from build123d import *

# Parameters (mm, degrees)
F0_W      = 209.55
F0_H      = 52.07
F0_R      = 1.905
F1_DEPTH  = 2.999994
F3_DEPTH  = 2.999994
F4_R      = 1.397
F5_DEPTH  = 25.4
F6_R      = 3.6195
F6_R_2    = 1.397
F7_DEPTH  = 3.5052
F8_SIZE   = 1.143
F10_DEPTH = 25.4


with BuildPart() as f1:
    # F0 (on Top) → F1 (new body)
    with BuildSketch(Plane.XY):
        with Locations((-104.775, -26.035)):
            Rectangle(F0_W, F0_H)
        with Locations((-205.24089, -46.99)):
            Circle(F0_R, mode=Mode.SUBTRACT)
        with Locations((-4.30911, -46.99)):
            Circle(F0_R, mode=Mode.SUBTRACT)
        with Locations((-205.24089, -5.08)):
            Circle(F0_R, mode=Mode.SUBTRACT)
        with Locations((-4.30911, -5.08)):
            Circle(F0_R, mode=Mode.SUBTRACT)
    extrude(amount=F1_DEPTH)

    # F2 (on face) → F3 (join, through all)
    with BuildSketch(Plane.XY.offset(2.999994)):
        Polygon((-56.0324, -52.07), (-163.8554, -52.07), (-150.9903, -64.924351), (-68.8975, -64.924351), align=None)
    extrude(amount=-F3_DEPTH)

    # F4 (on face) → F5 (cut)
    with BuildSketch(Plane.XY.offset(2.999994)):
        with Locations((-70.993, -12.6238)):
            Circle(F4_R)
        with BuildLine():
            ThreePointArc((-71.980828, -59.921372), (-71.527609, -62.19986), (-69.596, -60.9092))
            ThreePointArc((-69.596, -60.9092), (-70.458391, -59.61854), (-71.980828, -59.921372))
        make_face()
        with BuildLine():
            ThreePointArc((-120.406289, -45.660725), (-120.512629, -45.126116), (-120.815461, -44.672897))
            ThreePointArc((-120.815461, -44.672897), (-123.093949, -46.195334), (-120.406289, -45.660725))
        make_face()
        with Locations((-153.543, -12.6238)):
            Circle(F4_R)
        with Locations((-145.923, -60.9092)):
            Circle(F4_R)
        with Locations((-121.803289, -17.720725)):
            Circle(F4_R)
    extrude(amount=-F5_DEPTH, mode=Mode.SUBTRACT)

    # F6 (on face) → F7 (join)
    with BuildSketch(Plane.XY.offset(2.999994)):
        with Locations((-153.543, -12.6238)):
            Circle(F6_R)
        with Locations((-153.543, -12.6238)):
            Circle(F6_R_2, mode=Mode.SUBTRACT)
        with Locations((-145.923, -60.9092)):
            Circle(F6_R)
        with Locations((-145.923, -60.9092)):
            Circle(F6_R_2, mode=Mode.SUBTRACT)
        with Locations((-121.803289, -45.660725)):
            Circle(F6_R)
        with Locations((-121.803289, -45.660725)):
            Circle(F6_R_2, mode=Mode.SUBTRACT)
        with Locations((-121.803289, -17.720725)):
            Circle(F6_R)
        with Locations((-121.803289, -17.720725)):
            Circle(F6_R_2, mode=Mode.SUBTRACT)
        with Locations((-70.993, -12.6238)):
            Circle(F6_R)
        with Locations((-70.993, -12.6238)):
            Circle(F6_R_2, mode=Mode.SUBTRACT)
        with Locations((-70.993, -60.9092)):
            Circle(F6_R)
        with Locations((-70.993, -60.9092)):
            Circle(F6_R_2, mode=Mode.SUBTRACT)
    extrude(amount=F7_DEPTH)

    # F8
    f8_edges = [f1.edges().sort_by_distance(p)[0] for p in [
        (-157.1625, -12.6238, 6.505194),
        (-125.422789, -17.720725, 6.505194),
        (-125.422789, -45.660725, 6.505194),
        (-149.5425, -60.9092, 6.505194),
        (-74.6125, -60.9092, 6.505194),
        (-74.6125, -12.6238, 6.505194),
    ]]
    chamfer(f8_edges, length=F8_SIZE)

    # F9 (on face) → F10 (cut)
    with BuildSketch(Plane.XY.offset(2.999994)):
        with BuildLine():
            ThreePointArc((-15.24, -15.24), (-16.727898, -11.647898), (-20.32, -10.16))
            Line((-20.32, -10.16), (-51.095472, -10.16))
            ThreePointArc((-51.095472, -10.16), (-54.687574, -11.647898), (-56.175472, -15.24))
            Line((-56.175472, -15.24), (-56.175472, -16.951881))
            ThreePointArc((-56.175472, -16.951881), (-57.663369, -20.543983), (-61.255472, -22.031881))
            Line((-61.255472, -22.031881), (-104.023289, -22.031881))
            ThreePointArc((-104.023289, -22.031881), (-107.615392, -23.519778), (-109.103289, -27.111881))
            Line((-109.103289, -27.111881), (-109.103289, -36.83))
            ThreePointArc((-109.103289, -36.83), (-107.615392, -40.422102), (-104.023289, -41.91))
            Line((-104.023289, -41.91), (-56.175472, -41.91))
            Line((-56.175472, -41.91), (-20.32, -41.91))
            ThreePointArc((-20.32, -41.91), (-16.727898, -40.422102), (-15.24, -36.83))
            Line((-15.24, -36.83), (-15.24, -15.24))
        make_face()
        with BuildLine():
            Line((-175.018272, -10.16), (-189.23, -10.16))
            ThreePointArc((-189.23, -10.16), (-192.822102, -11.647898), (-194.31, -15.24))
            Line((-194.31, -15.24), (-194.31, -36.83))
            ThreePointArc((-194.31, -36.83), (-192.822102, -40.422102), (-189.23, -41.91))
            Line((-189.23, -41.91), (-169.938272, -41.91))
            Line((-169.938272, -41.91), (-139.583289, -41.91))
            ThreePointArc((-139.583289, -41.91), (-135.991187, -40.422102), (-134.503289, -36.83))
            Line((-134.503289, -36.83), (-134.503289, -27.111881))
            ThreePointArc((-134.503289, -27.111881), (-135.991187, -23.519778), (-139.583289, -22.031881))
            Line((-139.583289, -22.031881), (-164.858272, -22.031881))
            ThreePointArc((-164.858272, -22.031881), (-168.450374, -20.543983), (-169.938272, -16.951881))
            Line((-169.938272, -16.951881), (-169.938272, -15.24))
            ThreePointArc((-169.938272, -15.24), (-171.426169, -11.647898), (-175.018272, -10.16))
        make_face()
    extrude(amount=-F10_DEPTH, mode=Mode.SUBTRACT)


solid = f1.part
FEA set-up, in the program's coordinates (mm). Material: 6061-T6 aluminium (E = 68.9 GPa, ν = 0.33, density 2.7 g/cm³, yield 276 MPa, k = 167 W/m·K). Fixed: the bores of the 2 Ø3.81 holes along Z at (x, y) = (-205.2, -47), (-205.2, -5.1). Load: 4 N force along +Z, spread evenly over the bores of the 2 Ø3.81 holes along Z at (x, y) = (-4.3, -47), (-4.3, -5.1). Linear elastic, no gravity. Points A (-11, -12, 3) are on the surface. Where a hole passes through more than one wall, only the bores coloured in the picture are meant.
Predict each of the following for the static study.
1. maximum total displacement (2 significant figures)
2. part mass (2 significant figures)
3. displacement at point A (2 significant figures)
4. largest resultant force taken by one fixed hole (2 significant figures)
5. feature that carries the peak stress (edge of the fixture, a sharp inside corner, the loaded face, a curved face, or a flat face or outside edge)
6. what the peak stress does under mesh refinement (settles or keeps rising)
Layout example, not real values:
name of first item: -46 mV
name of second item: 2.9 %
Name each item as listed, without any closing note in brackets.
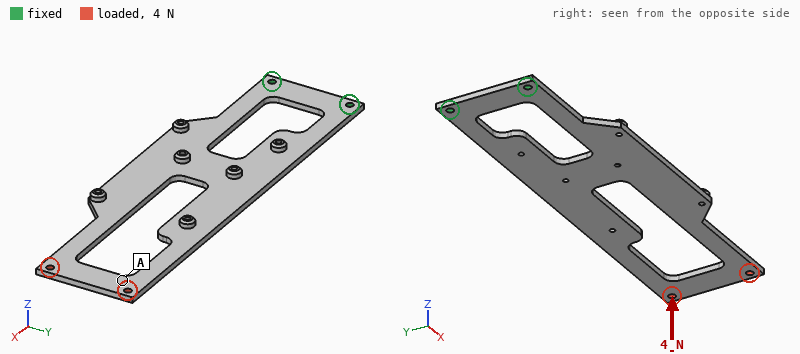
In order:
maximum total displacement: 2.4 mm
part mass: 69 g
displacement at point A: 2.2 mm
largest resultant force taken by one fixed hole: 2.1 N
feature that carries the peak stress: edge of the fixture
what the peak stress does under mesh refinement: keeps rising
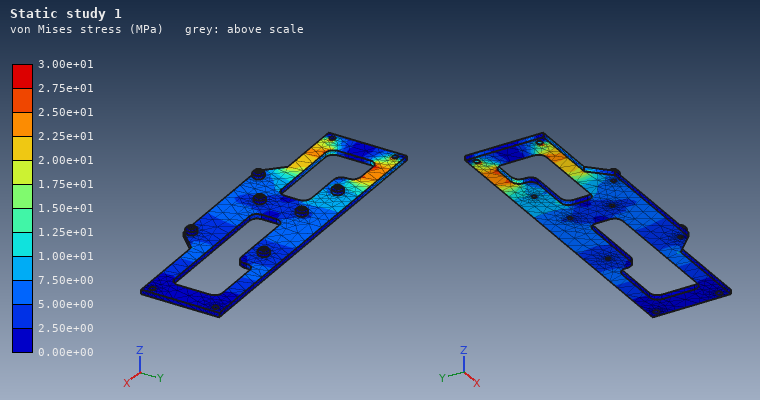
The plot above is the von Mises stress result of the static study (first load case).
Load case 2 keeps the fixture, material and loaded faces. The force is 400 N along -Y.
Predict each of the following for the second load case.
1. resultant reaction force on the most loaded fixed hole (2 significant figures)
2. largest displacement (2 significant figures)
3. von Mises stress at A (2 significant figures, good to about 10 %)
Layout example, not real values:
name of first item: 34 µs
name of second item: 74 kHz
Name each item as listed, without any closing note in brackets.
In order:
resultant reaction force on the most loaded fixed hole: 1.8 kN
largest displacement: 0.89 mm
von Mises stress at A: 25 MPa
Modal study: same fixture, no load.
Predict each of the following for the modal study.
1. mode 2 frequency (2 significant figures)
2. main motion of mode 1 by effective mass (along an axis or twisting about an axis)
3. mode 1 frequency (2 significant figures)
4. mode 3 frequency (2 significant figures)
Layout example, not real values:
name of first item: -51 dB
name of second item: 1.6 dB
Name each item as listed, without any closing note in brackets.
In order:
mode 2 frequency: 290 Hz
main motion of mode 1 by effective mass: along Z
mode 1 frequency: 52 Hz
mode 3 frequency: 340 Hz
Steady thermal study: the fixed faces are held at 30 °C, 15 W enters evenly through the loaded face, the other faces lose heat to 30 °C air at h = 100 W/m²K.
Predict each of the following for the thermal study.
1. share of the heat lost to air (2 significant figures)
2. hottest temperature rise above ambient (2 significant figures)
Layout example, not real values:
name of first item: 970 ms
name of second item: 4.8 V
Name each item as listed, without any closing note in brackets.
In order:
share of the heat lost to air: 99 %
hottest temperature rise above ambient: 43 K
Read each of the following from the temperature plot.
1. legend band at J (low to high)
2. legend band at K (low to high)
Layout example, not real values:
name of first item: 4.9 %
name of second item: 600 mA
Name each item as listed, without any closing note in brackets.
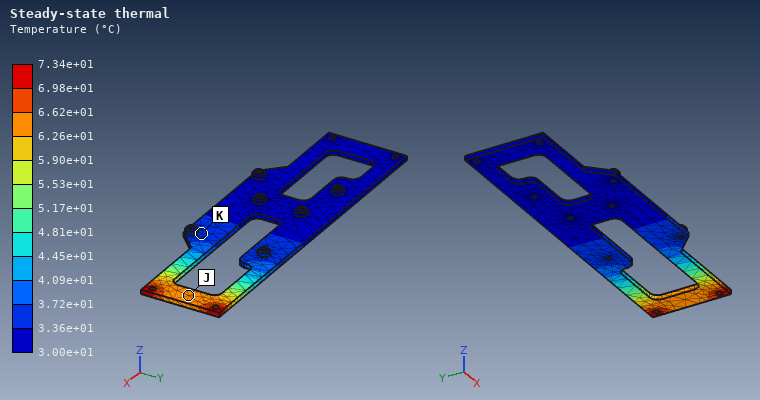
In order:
legend band at J: 6.26e+01 to 6.62e+01 °C
legend band at K: 3.36e+01 to 3.72e+01 °C
